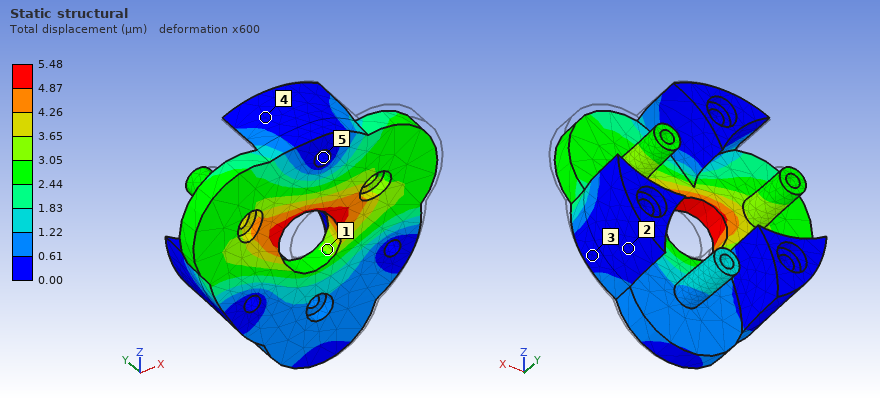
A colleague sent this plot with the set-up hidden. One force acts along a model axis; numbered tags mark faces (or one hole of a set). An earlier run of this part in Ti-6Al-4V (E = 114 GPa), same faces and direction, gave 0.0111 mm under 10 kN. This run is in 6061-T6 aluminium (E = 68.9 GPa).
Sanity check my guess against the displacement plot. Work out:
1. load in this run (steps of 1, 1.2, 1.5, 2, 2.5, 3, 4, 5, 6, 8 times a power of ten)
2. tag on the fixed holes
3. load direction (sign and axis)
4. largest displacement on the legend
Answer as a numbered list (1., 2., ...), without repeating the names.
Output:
1. 3 kN
2. 5
3. -X
4. 5.48 µm
